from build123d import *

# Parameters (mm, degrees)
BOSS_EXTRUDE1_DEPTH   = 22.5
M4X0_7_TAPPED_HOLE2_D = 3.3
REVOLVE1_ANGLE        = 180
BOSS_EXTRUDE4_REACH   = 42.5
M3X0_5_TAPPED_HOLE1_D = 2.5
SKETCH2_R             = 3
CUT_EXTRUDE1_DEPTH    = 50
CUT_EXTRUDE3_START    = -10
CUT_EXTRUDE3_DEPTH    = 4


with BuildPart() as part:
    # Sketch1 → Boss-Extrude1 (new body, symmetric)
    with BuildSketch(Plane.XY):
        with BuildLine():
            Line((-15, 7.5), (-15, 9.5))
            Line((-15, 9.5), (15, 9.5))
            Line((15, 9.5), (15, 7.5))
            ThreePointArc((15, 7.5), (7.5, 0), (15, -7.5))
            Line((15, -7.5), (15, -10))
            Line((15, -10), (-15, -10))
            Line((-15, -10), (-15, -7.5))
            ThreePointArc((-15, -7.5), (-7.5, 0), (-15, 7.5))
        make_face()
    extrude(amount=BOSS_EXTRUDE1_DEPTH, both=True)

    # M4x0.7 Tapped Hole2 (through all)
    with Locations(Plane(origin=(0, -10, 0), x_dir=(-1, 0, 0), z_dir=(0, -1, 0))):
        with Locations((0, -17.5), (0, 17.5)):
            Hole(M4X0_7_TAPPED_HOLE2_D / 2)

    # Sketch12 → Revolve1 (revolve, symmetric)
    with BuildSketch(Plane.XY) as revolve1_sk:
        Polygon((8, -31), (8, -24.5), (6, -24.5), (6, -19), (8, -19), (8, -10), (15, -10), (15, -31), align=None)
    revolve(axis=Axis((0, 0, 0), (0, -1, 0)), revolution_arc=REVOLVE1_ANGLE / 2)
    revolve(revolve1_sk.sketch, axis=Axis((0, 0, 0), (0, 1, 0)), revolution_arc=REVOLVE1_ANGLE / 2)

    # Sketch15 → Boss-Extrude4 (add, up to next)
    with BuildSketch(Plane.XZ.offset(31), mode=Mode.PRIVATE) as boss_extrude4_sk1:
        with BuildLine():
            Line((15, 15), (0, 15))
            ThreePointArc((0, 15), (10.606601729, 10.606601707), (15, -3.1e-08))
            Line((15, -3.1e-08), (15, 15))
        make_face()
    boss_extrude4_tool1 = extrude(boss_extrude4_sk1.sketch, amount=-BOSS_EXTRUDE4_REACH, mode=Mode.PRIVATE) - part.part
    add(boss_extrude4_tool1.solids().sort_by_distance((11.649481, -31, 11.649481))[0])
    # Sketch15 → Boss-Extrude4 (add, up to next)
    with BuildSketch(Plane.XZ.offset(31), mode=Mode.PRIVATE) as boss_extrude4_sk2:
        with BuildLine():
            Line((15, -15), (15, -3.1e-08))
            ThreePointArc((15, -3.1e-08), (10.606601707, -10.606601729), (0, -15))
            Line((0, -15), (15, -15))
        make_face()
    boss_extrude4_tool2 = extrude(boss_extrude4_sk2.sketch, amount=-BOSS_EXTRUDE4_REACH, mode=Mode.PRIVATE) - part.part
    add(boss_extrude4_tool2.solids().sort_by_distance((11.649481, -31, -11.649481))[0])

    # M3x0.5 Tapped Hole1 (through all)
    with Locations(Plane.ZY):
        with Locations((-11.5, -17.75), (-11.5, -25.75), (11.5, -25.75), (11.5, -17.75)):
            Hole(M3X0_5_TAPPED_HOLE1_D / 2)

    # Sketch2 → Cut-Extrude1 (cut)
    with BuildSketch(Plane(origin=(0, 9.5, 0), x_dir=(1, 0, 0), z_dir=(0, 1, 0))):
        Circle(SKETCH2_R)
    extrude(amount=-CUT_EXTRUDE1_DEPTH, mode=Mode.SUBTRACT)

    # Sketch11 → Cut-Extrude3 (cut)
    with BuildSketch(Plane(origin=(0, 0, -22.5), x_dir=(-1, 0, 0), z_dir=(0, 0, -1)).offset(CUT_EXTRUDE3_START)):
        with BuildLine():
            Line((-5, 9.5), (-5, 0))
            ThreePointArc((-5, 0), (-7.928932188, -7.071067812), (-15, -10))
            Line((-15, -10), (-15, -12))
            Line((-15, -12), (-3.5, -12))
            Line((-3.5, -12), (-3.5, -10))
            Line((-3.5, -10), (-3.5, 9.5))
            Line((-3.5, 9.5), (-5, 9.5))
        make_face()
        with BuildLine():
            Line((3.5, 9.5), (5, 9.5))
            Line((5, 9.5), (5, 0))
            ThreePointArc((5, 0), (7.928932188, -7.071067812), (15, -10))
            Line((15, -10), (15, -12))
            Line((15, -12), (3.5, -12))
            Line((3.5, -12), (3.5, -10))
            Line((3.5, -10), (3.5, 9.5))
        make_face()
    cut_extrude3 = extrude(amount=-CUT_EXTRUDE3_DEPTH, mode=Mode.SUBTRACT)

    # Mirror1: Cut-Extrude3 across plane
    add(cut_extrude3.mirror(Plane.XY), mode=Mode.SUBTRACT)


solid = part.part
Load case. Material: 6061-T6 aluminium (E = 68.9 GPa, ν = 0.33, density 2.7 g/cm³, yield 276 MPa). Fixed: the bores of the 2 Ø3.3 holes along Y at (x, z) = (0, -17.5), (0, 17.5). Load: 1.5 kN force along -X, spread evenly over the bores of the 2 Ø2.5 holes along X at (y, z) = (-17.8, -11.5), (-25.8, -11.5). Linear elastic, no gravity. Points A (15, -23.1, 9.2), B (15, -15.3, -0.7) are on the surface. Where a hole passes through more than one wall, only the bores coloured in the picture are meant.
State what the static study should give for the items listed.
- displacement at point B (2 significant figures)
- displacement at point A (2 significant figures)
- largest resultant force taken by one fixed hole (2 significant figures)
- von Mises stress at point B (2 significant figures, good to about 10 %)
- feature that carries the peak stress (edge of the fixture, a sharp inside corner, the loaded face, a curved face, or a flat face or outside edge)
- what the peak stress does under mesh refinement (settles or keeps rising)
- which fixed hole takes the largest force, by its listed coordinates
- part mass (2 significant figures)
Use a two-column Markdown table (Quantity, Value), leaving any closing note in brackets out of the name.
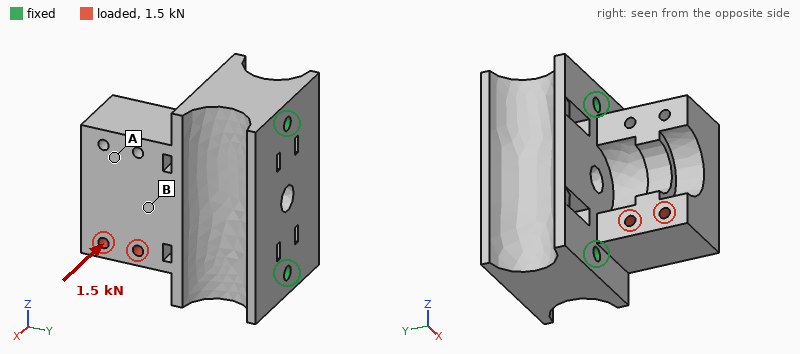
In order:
| Quantity | Value |
|---|---|
| displacement at point B | 22 µm |
| displacement at point A | 24 µm |
| largest resultant force taken by one fixed hole | 1.3 kN |
| von Mises stress at point B | 19 MPa |
| feature that carries the peak stress | edge of the fixture |
| what the peak stress does under mesh refinement | keeps rising |
| which fixed hole takes the largest force, by its listed coordinates | (0, -17.5) |
| part mass | 64 g |
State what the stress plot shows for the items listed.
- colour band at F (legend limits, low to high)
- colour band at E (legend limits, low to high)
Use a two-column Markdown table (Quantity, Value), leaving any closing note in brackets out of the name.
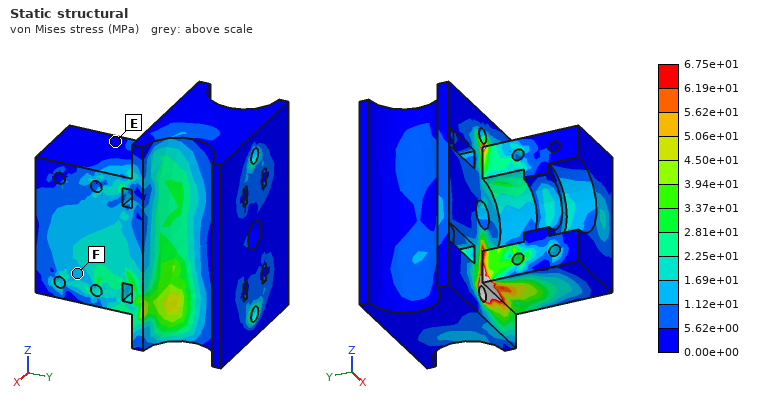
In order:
| Quantity | Value |
|---|---|
| colour band at F | 1.12e+01 to 1.69e+01 MPa |
| colour band at E | 0.00e+00 to 5.62e+00 MPa |
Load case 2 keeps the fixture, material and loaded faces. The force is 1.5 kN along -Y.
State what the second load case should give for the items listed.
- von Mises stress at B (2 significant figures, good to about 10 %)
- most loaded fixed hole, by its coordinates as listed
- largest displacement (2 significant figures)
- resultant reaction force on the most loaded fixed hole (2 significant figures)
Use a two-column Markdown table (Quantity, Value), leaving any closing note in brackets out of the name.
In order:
| Quantity | Value |
|---|---|
| von Mises stress at B | 3.6 MPa |
| most loaded fixed hole, by its coordinates as listed | (0, -17.5) |
| largest displacement | 16 µm |
| resultant reaction force on the most loaded fixed hole | 1.3 kN |
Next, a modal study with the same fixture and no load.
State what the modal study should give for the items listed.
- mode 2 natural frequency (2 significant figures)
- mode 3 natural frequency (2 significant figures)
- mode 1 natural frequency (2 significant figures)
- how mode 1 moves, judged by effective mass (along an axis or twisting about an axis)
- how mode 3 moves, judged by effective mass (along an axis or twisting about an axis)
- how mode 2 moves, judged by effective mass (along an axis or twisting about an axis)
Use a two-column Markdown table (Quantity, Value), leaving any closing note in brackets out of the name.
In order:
| Quantity | Value |
|---|---|
| mode 2 natural frequency | 14 kHz |
| mode 3 natural frequency | 20 kHz |
| mode 1 natural frequency | 8100 Hz |
| how mode 1 moves, judged by effective mass | along X |
| how mode 3 moves, judged by effective mass | along Z |
| how mode 2 moves, judged by effective mass | along Z |
